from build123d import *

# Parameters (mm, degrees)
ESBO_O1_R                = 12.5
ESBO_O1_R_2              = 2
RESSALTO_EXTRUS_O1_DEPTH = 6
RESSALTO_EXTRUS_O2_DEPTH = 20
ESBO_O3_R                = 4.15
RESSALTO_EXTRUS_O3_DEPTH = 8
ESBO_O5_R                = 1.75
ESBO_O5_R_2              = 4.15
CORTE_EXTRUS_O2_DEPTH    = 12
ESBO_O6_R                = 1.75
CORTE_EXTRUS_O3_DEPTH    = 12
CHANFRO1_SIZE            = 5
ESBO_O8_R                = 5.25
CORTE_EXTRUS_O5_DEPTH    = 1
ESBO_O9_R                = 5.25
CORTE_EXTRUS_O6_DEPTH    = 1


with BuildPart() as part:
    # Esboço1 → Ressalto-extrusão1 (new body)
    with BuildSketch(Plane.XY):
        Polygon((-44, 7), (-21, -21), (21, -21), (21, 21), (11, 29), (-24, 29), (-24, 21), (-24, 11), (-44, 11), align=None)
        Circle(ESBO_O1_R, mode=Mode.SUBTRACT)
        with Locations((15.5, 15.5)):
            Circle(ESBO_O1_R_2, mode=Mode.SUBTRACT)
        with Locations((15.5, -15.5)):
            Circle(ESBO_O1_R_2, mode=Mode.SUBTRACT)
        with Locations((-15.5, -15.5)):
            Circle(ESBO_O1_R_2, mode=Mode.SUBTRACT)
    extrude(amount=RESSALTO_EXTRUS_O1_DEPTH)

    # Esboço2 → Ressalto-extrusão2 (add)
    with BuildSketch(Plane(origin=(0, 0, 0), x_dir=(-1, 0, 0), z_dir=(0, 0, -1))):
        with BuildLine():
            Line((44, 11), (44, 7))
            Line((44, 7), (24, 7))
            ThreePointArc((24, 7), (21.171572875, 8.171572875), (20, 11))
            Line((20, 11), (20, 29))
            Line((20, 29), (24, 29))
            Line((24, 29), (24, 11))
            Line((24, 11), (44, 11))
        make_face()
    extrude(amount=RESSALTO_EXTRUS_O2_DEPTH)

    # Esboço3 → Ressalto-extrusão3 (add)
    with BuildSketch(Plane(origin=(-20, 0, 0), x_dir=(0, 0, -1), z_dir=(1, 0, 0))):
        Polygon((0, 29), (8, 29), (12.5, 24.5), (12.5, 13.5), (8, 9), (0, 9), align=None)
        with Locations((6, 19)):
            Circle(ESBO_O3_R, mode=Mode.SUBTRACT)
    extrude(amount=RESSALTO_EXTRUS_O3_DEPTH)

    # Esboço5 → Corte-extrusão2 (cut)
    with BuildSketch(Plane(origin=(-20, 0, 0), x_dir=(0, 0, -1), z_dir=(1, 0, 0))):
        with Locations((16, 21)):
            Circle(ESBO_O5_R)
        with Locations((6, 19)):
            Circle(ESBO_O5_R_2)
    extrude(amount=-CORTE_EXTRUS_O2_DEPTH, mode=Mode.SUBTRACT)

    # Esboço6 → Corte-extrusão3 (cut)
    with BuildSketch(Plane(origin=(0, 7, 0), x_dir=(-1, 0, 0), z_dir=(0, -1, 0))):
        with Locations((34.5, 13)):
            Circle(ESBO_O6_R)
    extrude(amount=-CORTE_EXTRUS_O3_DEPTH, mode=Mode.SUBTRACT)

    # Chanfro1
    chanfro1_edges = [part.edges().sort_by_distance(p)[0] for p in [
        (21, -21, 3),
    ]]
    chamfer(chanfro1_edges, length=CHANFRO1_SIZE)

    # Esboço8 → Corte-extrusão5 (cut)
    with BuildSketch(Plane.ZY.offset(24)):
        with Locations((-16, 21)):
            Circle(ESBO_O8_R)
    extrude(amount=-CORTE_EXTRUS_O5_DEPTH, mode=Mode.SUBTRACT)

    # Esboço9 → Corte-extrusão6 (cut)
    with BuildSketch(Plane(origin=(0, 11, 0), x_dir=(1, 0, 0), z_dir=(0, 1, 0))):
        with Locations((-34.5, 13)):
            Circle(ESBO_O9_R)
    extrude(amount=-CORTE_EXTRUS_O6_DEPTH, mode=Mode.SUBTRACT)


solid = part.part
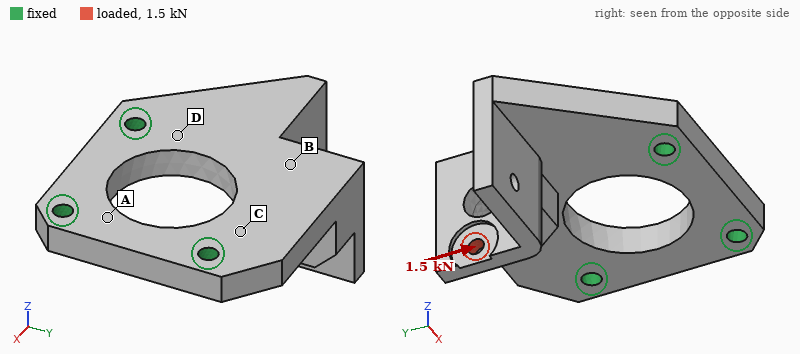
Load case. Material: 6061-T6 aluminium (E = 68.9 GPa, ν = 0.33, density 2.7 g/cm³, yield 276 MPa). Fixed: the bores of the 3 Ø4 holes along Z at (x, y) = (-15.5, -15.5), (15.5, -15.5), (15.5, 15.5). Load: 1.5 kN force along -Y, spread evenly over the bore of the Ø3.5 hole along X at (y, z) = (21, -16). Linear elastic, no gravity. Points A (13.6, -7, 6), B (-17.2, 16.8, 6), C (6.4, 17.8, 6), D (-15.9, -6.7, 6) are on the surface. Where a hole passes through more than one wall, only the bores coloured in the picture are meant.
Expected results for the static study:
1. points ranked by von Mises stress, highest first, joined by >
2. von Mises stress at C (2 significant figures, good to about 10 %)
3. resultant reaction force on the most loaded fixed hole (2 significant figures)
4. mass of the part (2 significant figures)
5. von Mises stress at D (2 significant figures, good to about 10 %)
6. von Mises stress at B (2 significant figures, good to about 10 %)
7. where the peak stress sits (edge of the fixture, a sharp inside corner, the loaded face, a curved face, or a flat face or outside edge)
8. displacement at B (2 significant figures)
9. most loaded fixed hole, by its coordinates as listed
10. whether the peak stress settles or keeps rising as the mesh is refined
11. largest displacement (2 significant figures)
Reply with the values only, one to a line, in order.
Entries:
C > D > B > A
110 MPa
1.5 kN
44 g
70 MPa
40 MPa
edge of the fixture
0.15 mm
(-15.5, -15.5)
keeps rising
0.43 mm
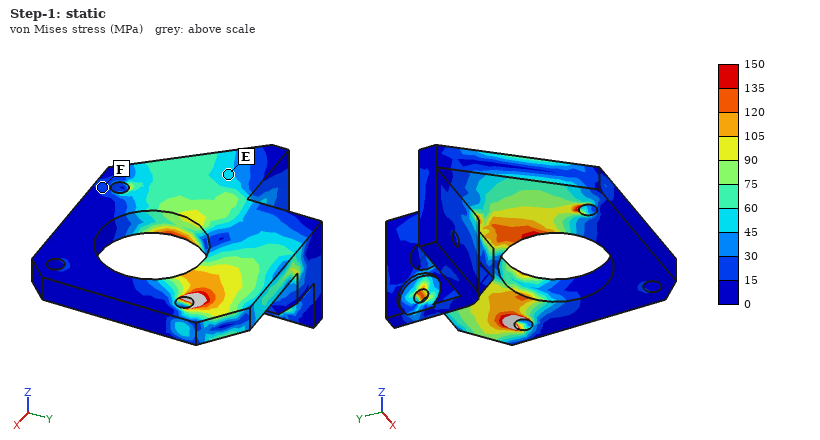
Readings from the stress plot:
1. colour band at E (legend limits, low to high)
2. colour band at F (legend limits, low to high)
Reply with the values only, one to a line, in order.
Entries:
45 to 60 MPa
15 to 30 MPa
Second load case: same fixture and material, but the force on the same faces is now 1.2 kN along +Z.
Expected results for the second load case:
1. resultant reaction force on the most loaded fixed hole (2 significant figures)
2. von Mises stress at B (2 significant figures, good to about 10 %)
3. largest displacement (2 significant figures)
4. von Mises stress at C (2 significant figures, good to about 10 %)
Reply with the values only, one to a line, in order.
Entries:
720 N
37 MPa
0.48 mm
120 MPa
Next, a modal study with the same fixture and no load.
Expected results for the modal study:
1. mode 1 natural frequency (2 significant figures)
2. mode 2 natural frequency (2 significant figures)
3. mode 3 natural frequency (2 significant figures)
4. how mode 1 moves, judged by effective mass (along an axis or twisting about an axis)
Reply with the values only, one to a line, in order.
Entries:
2300 Hz
5500 Hz
8100 Hz
along Z
